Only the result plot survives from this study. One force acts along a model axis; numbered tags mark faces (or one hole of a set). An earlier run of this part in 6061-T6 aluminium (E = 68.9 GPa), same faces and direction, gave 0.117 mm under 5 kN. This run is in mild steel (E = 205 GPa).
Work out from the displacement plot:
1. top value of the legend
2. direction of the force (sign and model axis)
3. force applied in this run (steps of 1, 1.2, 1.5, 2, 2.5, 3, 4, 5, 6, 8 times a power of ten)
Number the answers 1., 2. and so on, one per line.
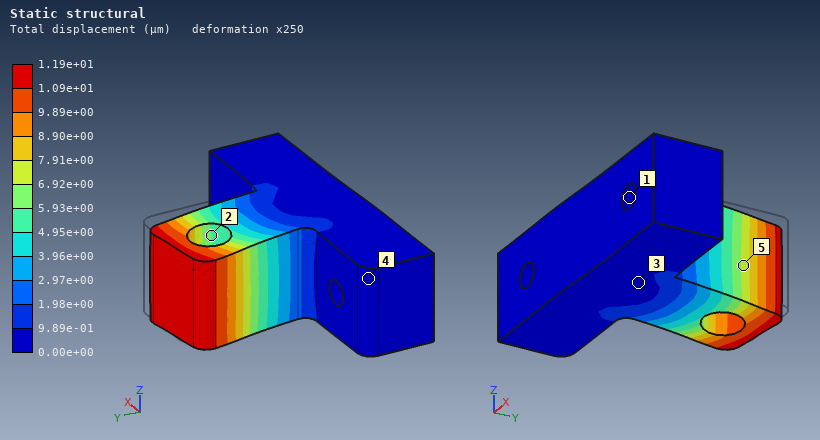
1. 1.19e+01 µm
2. -X
3. 1.5 kN
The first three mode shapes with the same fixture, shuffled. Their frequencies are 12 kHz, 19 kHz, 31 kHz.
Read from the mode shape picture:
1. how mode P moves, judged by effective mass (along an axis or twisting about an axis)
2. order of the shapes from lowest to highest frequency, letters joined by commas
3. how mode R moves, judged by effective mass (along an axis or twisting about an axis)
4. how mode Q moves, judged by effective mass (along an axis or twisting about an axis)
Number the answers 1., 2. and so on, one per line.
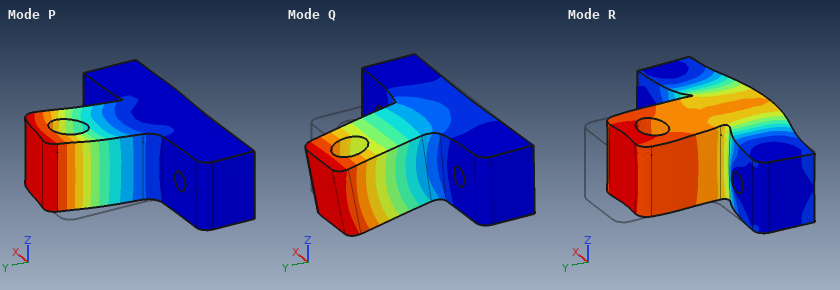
1. along X
2. Q, P, R
3. along Y
4. along Z
